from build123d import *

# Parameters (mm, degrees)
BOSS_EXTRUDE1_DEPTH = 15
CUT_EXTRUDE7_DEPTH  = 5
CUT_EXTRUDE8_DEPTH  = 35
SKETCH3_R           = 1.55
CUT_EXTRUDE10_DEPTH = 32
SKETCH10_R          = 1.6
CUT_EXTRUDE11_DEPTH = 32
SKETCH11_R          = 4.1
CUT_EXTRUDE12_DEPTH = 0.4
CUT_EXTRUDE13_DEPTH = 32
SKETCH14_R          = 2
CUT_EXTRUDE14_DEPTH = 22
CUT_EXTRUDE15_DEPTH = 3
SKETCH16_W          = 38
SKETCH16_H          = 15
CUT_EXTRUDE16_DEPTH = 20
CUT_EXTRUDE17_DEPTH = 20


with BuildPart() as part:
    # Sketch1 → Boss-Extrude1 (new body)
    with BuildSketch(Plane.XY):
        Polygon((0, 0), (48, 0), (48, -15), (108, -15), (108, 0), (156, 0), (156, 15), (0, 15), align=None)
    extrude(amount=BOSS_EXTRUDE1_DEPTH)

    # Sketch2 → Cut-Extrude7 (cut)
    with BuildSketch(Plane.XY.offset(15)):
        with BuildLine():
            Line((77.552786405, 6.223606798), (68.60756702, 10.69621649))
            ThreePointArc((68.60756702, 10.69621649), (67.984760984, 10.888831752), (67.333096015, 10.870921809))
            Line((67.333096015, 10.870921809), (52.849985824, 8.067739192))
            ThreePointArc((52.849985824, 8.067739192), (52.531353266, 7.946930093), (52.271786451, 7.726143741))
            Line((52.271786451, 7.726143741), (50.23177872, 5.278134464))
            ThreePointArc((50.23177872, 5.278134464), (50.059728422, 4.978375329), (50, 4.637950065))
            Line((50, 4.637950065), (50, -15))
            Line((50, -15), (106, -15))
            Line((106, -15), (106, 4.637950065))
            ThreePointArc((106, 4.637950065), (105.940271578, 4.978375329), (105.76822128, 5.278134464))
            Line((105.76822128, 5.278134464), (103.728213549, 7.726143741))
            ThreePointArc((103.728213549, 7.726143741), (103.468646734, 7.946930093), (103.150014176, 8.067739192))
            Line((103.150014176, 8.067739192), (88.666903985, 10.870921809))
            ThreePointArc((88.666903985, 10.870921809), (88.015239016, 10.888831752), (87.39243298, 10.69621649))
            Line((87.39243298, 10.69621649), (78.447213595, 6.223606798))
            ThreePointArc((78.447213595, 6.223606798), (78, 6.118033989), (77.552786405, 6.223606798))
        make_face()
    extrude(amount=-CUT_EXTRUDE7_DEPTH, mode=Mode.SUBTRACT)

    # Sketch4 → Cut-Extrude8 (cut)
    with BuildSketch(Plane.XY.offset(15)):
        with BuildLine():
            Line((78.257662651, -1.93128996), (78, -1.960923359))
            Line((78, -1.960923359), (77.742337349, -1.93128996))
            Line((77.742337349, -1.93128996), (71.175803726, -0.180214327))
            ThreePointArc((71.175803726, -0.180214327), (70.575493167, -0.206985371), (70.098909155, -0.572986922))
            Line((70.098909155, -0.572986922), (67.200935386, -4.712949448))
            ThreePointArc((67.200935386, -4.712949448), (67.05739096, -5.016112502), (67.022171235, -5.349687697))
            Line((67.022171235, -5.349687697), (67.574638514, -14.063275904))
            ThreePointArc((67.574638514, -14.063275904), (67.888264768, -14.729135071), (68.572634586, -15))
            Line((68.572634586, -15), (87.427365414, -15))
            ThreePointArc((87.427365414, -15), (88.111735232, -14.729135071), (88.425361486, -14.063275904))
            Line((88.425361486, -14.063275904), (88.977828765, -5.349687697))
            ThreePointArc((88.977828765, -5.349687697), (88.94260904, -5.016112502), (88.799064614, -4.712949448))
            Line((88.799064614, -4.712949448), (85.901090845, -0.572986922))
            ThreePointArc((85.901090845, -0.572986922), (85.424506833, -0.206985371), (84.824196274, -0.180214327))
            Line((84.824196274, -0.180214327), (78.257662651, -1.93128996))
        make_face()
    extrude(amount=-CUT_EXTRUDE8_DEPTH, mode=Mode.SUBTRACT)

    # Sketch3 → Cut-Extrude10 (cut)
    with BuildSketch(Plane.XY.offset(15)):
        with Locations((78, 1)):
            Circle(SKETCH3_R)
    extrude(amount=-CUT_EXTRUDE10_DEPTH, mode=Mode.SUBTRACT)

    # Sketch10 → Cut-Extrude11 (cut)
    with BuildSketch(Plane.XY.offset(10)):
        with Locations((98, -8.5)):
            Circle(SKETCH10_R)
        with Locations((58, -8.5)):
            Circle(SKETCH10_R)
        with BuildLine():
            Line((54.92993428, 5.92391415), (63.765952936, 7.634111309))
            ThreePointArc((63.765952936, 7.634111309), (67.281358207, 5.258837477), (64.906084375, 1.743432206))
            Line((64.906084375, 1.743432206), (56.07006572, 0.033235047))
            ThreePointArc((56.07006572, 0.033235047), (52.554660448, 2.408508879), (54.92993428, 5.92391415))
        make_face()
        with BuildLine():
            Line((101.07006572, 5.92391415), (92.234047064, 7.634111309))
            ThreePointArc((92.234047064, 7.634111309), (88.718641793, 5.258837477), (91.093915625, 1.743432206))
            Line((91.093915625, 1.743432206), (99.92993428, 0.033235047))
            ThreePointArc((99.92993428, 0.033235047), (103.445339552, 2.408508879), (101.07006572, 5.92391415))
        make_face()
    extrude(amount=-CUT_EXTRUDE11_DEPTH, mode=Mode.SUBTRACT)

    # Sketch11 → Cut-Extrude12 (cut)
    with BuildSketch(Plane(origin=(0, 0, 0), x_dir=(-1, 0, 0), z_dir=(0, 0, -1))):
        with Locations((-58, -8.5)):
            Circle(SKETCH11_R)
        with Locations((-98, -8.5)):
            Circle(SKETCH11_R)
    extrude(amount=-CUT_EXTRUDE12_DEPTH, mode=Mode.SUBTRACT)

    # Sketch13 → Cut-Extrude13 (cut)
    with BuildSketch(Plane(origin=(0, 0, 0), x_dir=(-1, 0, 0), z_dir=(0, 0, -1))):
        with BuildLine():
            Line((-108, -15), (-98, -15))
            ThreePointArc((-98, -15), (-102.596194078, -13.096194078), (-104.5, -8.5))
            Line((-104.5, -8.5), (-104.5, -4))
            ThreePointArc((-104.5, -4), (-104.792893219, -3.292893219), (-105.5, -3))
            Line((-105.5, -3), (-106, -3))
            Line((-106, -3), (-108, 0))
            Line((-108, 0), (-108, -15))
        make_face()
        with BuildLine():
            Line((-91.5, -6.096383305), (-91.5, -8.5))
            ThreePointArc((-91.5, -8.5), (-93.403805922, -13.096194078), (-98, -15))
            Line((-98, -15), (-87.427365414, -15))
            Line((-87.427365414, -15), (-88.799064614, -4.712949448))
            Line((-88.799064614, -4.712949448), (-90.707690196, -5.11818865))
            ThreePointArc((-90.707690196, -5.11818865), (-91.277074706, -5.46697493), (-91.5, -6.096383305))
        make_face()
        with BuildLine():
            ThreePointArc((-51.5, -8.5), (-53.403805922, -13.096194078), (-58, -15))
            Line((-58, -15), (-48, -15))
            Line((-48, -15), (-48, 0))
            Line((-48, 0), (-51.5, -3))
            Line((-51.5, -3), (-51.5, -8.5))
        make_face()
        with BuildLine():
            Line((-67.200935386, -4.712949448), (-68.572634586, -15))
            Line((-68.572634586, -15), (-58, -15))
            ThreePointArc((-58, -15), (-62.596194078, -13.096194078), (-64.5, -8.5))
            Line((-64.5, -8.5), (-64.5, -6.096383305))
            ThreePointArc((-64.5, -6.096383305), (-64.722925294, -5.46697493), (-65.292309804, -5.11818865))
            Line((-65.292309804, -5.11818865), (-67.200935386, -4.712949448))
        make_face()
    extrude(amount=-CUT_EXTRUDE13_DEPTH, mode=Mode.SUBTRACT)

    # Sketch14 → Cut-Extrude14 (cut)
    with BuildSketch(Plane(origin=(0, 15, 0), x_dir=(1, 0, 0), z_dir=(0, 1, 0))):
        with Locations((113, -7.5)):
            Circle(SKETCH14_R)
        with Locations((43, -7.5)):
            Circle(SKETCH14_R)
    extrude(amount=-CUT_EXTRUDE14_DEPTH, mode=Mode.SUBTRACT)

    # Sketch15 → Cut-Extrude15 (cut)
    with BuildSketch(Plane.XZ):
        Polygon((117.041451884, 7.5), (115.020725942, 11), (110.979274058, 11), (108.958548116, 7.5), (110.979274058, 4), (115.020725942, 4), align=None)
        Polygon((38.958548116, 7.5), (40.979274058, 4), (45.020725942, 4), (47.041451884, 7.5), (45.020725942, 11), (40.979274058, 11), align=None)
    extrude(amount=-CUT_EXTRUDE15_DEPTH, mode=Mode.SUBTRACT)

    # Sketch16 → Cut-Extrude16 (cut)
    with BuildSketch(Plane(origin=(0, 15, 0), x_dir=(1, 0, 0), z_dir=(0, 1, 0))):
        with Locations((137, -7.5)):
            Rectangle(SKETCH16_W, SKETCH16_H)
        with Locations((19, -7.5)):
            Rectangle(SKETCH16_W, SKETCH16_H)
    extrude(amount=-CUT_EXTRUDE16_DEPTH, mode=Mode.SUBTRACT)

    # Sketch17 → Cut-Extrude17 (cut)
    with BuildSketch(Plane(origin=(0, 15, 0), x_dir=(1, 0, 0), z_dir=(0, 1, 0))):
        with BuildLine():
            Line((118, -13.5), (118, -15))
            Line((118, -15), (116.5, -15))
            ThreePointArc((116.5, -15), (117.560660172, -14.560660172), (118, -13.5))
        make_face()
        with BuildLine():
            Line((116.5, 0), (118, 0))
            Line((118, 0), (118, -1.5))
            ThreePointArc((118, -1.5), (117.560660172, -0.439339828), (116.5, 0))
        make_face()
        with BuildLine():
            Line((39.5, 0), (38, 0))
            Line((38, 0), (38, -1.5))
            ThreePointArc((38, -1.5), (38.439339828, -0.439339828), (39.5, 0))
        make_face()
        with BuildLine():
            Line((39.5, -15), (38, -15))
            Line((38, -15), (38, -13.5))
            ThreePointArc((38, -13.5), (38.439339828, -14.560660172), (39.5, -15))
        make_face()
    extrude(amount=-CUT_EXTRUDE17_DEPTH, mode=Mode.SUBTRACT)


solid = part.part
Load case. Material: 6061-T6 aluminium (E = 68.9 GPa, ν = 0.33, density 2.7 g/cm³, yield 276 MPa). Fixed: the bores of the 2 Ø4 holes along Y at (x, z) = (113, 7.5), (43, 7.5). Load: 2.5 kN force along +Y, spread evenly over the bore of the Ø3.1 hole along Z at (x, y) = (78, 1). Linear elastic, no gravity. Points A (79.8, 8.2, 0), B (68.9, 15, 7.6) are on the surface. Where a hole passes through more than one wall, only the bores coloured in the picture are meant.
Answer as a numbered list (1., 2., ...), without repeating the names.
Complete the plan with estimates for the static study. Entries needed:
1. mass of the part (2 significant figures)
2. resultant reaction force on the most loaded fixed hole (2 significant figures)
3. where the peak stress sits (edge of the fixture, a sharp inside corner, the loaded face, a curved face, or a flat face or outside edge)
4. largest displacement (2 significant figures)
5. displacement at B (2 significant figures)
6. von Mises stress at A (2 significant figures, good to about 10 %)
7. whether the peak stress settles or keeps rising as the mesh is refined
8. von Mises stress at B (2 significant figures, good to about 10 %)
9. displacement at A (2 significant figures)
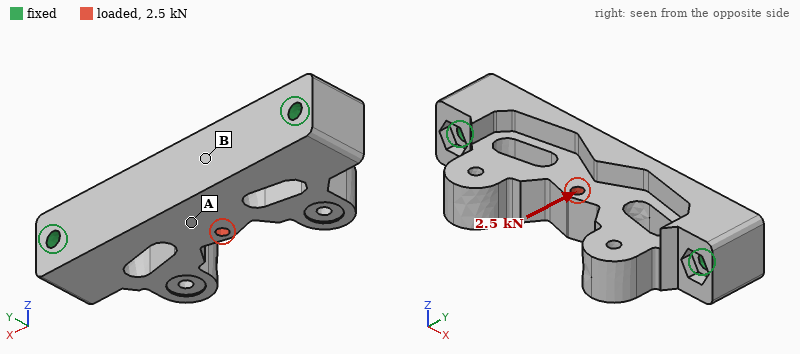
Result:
1. 47 g
2. 1.3 kN
3. edge of the fixture
4. 52 µm
5. 40 µm
6. 15 MPa
7. keeps rising
8. 44 MPa
9. 49 µm
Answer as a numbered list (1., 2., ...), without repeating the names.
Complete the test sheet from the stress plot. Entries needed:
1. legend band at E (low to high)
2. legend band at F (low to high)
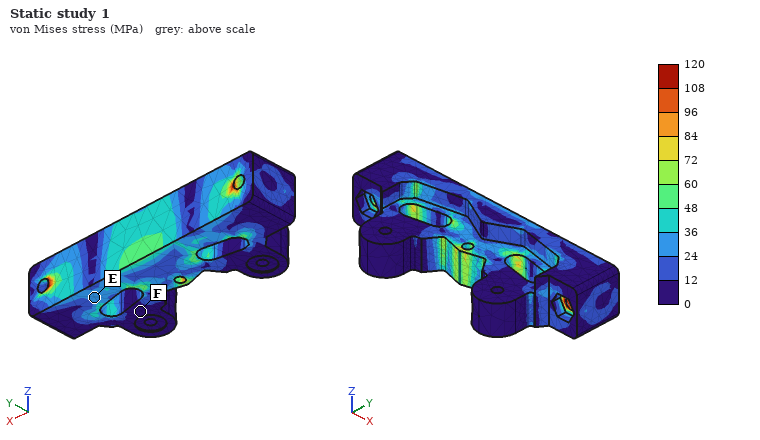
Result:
1. 24 to 36 MPa
2. 0 to 12 MPa
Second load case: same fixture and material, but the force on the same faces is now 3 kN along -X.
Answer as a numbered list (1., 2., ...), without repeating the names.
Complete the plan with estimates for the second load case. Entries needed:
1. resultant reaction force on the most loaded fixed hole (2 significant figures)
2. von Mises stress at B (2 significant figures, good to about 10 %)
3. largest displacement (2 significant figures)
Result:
1. 1.6 kN
2. 9.8 MPa
3. 14 µm
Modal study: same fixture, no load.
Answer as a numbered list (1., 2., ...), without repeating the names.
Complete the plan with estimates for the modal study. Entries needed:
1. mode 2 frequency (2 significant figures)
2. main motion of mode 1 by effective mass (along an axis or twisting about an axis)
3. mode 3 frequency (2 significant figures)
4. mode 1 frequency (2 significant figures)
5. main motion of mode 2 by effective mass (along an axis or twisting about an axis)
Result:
1. 8700 Hz
2. along Z
3. 12 kHz
4. 7800 Hz
5. along Y
